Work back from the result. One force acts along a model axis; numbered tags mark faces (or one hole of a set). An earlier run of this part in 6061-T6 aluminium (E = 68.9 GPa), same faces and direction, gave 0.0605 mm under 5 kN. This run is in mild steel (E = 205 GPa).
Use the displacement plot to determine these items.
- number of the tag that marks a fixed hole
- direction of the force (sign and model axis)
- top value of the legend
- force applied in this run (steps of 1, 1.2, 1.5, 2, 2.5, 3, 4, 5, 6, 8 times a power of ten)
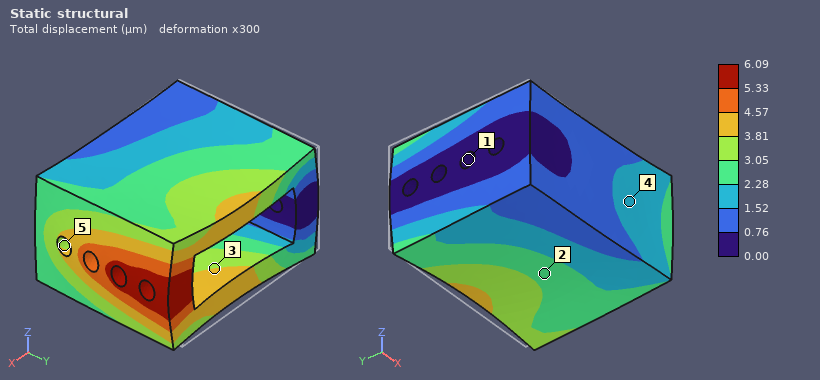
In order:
1
+X
6.09 µm
1.5 kN
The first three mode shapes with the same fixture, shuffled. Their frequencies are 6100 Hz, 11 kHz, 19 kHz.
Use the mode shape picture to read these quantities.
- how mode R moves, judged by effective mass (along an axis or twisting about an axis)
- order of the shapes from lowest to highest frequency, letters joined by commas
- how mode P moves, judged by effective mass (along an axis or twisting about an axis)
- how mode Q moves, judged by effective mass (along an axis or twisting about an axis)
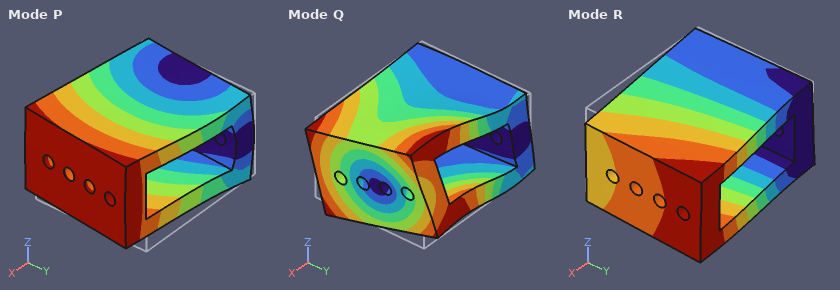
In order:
along Z
R, P, Q
along Y
twisting about X
